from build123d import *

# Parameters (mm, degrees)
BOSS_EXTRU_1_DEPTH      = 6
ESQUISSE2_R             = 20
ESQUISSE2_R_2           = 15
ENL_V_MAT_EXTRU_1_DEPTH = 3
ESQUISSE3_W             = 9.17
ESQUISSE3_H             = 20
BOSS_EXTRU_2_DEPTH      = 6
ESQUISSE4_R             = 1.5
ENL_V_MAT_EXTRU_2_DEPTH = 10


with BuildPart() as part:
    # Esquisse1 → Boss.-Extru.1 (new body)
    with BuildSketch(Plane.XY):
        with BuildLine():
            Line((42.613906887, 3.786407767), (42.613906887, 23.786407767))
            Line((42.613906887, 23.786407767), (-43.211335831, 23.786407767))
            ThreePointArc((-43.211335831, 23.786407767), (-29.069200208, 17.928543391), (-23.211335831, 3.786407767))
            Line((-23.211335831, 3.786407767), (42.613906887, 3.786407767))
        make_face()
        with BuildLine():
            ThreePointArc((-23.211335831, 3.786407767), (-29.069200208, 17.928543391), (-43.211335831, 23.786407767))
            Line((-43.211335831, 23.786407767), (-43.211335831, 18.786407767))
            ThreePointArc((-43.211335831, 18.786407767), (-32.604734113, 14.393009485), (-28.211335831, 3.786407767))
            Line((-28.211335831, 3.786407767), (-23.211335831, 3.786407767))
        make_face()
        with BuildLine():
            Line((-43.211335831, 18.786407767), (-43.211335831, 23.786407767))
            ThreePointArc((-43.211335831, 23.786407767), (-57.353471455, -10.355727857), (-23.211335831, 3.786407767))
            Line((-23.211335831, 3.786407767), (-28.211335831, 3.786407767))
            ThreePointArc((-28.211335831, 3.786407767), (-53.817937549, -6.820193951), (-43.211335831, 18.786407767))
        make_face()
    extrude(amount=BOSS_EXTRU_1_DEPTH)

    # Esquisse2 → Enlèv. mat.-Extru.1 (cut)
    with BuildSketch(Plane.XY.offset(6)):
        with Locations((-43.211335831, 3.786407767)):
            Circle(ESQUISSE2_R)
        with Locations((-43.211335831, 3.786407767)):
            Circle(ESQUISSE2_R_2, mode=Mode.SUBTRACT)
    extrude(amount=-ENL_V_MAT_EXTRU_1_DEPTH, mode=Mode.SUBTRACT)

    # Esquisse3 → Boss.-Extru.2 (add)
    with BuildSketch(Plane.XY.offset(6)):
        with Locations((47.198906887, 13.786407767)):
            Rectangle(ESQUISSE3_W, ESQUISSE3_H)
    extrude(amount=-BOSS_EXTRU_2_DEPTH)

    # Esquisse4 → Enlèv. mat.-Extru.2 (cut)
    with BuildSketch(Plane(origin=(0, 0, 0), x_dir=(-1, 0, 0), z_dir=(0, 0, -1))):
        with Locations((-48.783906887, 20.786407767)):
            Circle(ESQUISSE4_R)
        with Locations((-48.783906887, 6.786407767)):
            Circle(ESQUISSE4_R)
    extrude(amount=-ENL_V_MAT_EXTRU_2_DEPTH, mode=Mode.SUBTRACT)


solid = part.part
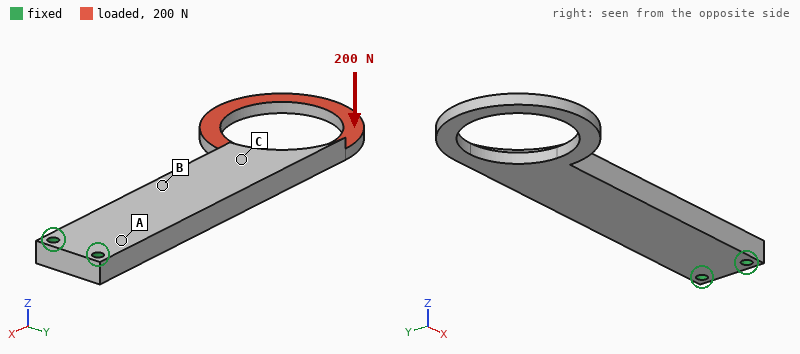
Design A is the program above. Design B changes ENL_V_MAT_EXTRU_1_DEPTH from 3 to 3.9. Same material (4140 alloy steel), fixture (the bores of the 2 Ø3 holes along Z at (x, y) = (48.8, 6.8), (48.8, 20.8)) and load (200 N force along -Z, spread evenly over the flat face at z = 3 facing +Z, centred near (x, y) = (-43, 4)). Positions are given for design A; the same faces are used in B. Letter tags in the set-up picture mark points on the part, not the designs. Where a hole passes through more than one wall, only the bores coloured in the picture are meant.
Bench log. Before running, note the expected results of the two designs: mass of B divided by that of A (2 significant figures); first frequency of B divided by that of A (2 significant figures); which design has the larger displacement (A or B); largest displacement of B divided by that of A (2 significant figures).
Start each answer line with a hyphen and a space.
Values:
- 0.96
- 1.1
- B
- 1.4
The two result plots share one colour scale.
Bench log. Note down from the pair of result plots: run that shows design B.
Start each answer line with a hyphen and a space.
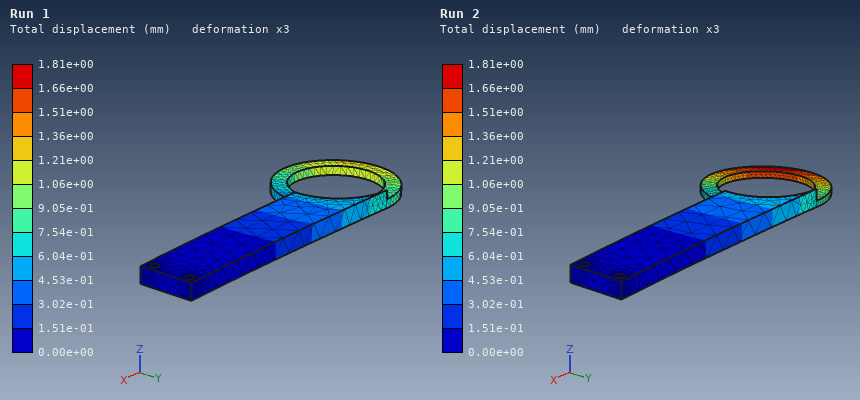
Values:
- Run 2
